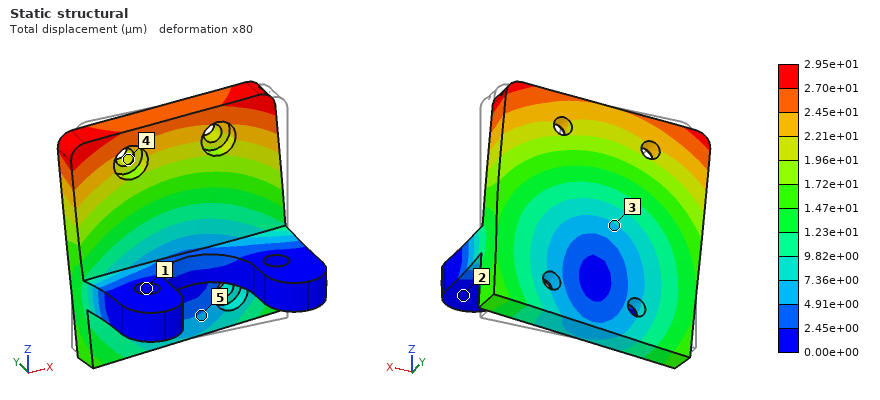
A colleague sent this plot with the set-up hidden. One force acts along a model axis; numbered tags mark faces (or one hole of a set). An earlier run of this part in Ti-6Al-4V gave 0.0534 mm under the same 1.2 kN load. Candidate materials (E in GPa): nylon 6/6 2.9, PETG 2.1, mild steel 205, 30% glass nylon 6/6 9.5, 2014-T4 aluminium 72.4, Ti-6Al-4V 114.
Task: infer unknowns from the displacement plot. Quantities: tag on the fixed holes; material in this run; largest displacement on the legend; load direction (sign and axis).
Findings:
1
mild steel
2.95e+01 µm
-X
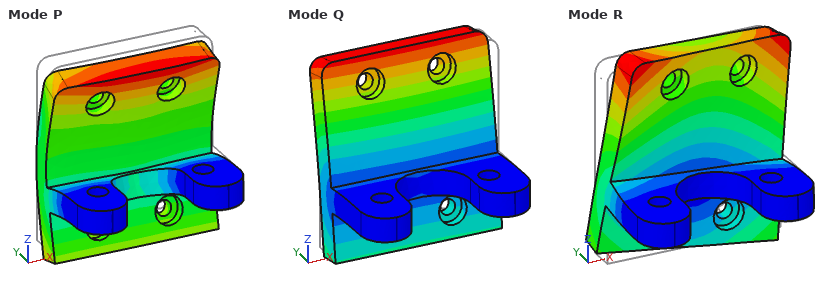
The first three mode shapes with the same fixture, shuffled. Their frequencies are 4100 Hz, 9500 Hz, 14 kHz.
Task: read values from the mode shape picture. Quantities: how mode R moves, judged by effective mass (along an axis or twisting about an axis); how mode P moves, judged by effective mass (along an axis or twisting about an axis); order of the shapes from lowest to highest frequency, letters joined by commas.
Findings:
along X
along Z
Q, R, P
